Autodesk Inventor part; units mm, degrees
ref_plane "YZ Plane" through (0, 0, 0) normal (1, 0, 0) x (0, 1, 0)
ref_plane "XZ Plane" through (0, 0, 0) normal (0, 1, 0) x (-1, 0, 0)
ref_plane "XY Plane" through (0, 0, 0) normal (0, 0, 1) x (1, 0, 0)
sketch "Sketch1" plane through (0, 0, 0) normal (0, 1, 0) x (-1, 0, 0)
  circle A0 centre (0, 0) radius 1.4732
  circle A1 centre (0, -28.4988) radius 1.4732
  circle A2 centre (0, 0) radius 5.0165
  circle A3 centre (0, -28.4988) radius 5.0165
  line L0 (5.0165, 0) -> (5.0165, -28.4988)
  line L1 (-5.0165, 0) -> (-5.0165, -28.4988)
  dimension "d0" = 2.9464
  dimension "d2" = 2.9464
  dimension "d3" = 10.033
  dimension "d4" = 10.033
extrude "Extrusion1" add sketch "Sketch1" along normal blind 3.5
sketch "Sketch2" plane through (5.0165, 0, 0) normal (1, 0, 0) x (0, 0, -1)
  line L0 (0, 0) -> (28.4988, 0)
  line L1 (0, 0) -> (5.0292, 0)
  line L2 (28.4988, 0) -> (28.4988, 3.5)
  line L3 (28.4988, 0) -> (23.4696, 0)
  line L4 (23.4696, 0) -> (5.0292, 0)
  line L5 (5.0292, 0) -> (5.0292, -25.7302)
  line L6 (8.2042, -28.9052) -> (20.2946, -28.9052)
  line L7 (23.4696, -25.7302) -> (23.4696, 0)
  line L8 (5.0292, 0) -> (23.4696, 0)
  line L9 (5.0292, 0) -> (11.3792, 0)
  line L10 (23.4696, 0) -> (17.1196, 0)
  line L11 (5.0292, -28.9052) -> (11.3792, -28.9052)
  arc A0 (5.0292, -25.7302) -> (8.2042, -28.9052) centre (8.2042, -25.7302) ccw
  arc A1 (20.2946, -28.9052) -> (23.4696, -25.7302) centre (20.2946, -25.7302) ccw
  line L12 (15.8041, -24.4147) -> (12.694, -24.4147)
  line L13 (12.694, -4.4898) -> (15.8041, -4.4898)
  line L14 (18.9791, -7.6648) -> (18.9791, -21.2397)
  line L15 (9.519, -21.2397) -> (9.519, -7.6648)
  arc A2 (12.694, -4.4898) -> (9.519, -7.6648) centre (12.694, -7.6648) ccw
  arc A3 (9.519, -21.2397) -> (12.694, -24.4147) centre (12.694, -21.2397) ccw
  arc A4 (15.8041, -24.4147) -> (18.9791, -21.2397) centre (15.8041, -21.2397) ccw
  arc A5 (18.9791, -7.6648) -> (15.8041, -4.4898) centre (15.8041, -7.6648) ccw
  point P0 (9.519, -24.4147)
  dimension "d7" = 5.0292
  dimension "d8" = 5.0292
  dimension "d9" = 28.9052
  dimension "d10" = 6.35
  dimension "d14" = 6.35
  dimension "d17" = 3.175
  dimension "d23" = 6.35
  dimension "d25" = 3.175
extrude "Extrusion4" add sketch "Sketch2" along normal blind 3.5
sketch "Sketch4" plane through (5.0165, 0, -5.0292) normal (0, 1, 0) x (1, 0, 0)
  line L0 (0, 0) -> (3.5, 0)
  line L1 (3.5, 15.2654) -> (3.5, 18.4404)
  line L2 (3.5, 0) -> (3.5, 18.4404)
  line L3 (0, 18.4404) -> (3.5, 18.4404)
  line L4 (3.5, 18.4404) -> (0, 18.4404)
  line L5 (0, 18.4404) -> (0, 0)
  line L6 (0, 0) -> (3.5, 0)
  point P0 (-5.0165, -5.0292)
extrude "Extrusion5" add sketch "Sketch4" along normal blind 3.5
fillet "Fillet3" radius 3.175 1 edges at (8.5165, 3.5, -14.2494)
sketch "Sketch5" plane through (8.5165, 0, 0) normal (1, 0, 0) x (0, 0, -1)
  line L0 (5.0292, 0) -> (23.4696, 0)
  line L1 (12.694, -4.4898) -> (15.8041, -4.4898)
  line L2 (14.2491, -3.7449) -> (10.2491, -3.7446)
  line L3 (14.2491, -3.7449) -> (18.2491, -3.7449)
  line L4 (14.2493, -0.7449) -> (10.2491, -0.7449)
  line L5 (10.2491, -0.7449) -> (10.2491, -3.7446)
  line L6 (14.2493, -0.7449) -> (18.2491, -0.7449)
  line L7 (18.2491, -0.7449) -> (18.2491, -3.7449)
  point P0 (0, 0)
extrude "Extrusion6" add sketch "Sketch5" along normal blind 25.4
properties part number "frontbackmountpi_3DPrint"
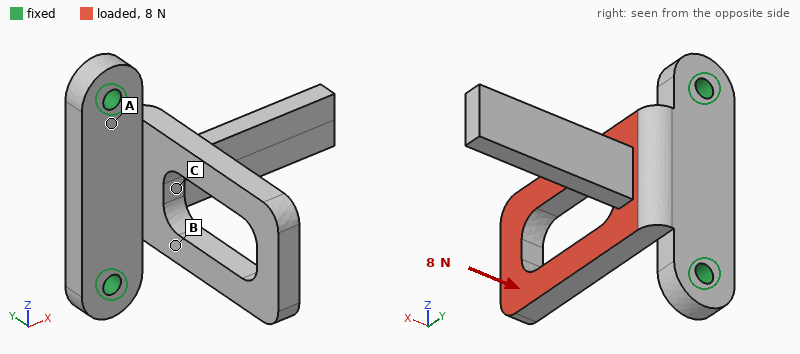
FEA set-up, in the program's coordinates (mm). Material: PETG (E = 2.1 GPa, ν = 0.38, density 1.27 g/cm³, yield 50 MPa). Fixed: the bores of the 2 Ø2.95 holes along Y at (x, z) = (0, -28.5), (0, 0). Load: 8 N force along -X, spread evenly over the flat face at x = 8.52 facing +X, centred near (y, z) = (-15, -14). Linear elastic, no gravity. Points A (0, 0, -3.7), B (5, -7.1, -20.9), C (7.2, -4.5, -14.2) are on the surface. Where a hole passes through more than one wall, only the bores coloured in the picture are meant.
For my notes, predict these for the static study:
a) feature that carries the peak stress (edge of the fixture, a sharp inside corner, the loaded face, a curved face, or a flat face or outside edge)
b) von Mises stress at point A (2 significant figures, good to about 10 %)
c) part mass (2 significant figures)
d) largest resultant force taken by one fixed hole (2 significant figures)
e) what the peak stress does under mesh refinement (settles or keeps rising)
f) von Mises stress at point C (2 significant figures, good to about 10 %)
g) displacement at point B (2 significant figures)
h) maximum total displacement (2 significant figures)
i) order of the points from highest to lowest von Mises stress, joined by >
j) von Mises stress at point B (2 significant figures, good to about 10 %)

a sharp inside corner
2.7 MPa
4.1 g
4.3 N
keeps rising
0.78 MPa
0.11 mm
0.62 mm
B > A > C
3.6 MPa
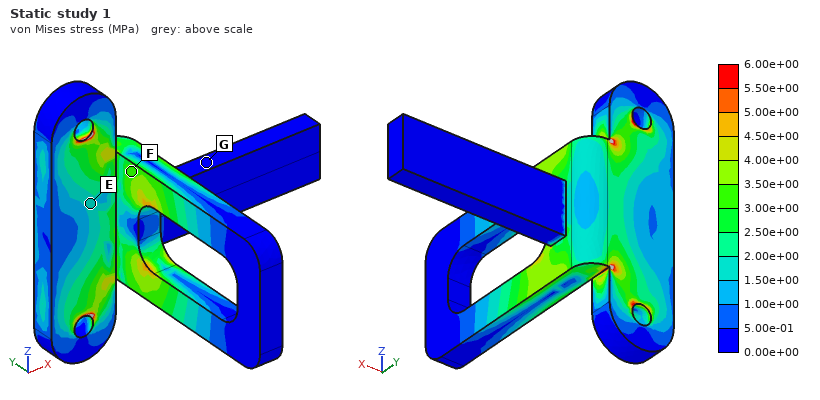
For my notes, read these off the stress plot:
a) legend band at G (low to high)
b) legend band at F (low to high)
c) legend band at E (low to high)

0.00e+00 to 5.00e-01 MPa
3.00e+00 to 3.50e+00 MPa
1.50e+00 to 2.00e+00 MPa
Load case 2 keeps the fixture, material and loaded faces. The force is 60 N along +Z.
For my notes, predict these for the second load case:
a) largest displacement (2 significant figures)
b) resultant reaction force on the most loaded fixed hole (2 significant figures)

0.68 mm
58 N
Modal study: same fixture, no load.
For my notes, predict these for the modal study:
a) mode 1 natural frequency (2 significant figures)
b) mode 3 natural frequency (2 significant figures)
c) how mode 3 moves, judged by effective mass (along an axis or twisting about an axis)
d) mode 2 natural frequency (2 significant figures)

490 Hz
1400 Hz
along Z
860 Hz
